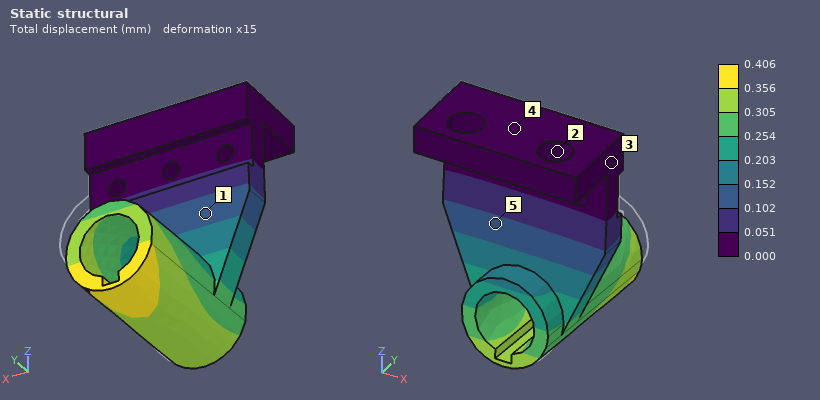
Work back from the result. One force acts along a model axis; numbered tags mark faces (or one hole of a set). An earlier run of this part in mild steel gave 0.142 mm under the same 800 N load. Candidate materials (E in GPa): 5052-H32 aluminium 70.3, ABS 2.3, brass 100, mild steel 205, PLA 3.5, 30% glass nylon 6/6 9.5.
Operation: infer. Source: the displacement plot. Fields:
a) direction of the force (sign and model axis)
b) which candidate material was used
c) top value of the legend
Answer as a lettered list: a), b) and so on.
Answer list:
a) -Y
b) 5052-H32 aluminium
c) 0.406 mm
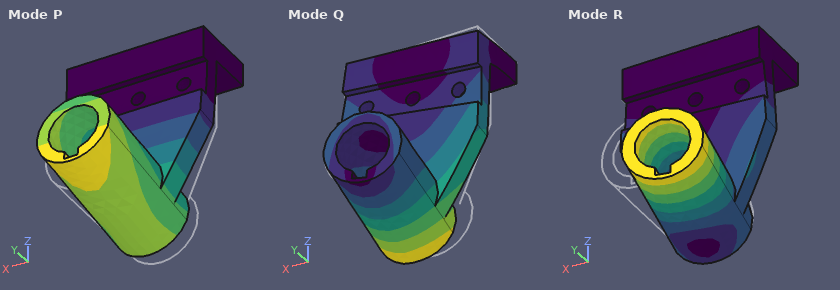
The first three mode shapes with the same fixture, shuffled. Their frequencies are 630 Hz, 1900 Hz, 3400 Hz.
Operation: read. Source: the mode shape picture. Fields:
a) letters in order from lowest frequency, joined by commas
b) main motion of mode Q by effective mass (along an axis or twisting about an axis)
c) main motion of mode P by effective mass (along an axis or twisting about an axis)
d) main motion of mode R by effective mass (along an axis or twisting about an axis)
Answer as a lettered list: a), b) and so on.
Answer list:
a) P, R, Q
b) along X
c) along Y
d) along X
